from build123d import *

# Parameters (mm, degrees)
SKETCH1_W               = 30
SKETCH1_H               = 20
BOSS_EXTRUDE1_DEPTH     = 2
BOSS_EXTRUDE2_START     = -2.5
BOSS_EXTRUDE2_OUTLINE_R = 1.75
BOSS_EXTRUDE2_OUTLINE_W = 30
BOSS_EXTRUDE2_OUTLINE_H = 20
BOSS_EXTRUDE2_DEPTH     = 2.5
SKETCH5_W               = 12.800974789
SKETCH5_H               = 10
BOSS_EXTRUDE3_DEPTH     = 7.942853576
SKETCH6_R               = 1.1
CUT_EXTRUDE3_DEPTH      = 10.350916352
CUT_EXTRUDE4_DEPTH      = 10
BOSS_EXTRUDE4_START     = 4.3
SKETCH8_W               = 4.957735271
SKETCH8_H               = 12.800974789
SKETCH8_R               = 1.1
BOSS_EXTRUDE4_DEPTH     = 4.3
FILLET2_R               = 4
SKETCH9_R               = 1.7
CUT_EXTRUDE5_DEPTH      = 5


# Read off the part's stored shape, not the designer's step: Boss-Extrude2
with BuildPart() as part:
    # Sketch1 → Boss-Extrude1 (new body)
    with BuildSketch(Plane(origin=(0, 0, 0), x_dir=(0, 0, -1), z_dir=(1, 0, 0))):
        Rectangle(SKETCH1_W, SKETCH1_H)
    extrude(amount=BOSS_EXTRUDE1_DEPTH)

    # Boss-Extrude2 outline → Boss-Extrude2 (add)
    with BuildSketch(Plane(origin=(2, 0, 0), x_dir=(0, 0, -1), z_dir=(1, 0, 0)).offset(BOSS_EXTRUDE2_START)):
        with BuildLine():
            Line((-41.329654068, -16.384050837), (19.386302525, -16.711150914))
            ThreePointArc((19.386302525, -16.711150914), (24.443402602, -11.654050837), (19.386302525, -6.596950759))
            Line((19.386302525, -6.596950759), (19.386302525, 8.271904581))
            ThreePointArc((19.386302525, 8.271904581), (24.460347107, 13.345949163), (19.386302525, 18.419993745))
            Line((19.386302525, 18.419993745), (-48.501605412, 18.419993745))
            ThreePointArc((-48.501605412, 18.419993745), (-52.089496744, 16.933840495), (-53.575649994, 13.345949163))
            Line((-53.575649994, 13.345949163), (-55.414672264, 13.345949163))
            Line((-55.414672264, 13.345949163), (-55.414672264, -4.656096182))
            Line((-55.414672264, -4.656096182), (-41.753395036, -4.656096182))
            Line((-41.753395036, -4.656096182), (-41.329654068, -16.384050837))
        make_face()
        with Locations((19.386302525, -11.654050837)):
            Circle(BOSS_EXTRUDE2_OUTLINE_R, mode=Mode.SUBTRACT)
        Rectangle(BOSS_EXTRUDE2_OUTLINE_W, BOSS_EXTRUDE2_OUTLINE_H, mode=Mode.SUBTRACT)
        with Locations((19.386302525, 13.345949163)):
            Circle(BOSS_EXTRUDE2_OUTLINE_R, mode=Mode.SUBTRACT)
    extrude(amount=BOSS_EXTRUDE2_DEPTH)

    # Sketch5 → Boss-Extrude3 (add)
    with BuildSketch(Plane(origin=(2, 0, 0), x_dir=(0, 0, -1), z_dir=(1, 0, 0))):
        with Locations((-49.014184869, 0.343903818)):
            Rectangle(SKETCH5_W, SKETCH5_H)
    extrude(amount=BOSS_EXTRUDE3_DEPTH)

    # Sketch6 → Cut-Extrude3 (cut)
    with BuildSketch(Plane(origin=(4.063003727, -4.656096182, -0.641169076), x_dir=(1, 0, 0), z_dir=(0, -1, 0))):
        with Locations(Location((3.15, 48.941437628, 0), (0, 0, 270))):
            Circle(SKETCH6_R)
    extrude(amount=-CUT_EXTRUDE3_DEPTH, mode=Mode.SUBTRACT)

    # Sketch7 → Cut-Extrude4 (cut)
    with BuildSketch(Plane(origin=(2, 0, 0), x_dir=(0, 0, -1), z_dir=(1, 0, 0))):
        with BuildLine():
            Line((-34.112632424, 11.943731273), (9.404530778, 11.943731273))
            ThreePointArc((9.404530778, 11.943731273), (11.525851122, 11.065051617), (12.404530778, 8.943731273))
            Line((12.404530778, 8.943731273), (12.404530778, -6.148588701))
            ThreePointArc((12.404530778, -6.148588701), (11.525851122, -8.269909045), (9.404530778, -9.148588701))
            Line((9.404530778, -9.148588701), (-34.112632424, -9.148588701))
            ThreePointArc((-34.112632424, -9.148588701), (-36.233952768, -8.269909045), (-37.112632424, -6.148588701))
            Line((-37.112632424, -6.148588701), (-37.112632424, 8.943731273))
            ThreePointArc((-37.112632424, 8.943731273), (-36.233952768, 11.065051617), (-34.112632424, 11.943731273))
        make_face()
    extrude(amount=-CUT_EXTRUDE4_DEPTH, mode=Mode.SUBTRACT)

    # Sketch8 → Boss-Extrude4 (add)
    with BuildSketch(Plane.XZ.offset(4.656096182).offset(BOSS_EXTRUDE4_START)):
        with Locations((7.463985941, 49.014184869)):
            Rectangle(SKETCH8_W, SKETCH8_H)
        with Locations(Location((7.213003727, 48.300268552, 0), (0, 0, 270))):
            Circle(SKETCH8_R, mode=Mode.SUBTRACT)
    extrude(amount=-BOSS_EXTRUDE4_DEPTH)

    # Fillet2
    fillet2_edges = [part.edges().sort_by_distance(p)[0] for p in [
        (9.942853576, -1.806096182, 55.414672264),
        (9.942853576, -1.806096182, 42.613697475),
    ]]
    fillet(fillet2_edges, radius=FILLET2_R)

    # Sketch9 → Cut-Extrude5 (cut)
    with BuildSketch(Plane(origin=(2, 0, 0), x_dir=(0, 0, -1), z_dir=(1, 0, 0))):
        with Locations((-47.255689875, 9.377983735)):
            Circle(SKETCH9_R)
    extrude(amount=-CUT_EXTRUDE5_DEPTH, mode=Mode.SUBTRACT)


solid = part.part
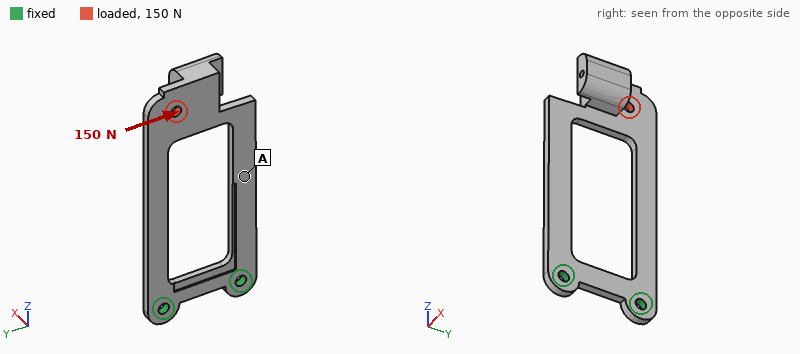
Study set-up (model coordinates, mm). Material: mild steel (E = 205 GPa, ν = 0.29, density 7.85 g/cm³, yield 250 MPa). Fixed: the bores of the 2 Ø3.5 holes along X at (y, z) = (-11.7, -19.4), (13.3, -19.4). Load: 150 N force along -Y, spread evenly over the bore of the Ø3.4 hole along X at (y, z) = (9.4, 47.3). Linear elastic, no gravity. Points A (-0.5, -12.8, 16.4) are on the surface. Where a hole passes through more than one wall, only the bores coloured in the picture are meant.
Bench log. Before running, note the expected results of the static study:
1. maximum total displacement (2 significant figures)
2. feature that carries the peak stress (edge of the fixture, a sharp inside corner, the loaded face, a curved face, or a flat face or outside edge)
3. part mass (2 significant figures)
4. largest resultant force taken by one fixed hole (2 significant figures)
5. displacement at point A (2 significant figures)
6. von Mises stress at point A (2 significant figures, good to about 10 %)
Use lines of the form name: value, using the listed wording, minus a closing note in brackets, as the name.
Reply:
maximum total displacement: 97 µm
feature that carries the peak stress: a curved face
part mass: 37 g
largest resultant force taken by one fixed hole: 290 N
displacement at point A: 52 µm
von Mises stress at point A: 15 MPa
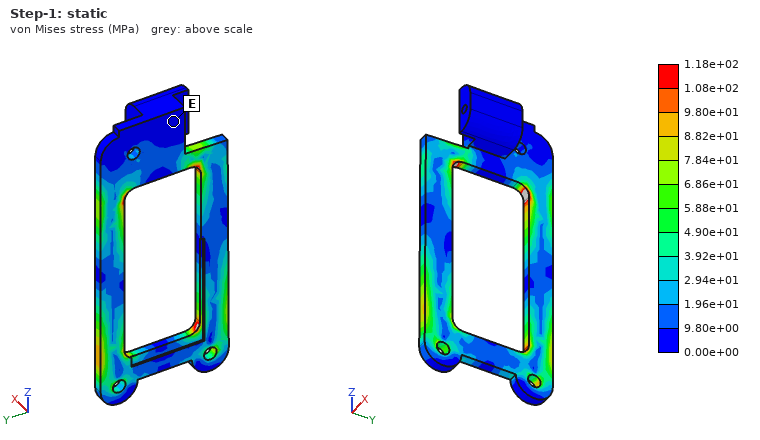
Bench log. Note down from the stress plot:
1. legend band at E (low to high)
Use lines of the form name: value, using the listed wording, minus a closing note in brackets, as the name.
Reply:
legend band at E: 0.00e+00 to 9.80e+00 MPa
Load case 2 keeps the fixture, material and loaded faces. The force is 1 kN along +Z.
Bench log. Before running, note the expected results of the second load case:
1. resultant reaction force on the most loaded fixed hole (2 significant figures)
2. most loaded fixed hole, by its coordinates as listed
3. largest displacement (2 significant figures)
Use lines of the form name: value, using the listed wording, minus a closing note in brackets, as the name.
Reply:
resultant reaction force on the most loaded fixed hole: 800 N
most loaded fixed hole, by its coordinates as listed: (13.3, -19.4)
largest displacement: 26 µm
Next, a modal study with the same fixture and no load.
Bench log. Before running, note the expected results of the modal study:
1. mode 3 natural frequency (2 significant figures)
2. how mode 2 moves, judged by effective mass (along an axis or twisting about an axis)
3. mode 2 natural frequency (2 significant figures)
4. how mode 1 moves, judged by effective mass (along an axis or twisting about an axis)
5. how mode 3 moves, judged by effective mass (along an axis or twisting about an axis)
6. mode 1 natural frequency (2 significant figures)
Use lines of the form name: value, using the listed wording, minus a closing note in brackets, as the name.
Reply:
mode 3 natural frequency: 1400 Hz
how mode 2 moves, judged by effective mass: along Y
mode 2 natural frequency: 1100 Hz
how mode 1 moves, judged by effective mass: along X
how mode 3 moves, judged by effective mass: along Y
mode 1 natural frequency: 230 Hz
